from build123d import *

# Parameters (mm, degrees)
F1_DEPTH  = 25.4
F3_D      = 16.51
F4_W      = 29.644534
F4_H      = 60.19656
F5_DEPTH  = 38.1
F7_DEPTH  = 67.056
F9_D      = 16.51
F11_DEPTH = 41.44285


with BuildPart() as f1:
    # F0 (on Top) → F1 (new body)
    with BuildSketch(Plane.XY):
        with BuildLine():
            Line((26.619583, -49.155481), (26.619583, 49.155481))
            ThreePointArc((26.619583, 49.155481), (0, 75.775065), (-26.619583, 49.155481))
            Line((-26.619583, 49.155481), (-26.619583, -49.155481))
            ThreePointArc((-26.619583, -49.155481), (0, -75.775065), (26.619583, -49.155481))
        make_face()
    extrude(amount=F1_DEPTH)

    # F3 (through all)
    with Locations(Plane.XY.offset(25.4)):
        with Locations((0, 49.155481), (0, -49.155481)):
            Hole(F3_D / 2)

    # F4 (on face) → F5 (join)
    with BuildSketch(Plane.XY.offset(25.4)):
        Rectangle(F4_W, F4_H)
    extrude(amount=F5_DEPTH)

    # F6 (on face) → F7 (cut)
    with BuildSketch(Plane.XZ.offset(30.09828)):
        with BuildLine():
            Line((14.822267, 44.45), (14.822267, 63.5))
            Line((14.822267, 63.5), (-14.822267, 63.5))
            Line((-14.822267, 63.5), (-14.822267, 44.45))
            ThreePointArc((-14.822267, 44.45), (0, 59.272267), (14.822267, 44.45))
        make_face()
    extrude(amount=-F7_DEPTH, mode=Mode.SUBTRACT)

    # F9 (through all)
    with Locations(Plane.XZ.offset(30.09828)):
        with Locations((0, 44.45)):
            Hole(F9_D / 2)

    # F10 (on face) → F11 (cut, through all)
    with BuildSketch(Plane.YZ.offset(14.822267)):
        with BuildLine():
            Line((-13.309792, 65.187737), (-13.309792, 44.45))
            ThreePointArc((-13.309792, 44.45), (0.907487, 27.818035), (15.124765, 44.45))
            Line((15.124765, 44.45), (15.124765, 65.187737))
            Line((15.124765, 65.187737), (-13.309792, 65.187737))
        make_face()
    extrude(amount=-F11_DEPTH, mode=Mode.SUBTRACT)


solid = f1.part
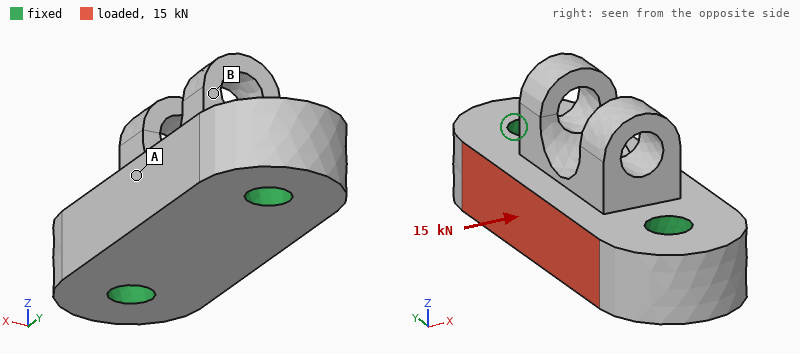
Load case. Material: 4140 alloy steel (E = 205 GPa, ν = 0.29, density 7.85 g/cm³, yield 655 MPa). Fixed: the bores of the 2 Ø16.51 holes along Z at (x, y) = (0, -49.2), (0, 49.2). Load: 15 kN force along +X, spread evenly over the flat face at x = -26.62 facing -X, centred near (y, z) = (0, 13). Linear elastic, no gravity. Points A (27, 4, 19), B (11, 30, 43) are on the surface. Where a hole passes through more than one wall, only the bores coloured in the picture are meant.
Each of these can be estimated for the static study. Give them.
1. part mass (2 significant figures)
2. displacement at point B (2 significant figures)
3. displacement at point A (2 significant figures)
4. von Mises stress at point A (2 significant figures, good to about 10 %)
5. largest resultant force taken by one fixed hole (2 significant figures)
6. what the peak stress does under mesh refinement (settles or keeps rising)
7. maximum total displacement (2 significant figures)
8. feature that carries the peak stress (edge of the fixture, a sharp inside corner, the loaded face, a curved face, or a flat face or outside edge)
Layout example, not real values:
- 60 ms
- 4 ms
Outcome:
- 1.6 kg
- 1.9 µm
- 2.3 µm
- 8.7 MPa
- 7.6 kN
- keeps rising
- 3.3 µm
- edge of the fixture
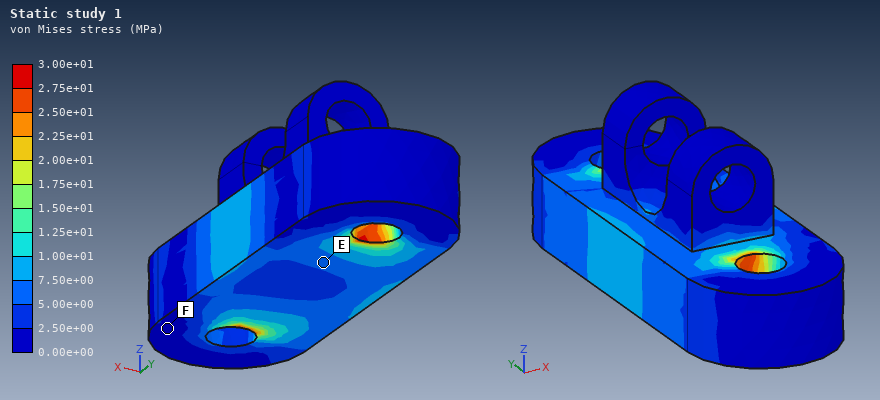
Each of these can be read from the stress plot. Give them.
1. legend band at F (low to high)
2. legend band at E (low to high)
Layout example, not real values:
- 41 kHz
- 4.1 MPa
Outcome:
- 0.00e+00 to 2.50e+00 MPa
- 5.00e+00 to 7.50e+00 MPa
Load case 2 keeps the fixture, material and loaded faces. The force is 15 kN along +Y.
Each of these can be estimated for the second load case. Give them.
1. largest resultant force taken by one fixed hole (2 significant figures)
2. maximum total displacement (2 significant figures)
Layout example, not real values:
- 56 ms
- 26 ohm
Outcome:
- 8.2 kN
- 2.1 µm
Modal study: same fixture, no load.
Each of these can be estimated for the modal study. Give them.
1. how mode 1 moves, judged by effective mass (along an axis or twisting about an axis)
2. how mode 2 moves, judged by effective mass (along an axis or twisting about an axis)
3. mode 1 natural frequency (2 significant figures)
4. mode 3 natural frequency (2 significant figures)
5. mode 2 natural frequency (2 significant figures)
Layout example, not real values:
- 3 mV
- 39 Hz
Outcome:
- along X
- along Z
- 8300 Hz
- 12 kHz
- 9200 Hz
